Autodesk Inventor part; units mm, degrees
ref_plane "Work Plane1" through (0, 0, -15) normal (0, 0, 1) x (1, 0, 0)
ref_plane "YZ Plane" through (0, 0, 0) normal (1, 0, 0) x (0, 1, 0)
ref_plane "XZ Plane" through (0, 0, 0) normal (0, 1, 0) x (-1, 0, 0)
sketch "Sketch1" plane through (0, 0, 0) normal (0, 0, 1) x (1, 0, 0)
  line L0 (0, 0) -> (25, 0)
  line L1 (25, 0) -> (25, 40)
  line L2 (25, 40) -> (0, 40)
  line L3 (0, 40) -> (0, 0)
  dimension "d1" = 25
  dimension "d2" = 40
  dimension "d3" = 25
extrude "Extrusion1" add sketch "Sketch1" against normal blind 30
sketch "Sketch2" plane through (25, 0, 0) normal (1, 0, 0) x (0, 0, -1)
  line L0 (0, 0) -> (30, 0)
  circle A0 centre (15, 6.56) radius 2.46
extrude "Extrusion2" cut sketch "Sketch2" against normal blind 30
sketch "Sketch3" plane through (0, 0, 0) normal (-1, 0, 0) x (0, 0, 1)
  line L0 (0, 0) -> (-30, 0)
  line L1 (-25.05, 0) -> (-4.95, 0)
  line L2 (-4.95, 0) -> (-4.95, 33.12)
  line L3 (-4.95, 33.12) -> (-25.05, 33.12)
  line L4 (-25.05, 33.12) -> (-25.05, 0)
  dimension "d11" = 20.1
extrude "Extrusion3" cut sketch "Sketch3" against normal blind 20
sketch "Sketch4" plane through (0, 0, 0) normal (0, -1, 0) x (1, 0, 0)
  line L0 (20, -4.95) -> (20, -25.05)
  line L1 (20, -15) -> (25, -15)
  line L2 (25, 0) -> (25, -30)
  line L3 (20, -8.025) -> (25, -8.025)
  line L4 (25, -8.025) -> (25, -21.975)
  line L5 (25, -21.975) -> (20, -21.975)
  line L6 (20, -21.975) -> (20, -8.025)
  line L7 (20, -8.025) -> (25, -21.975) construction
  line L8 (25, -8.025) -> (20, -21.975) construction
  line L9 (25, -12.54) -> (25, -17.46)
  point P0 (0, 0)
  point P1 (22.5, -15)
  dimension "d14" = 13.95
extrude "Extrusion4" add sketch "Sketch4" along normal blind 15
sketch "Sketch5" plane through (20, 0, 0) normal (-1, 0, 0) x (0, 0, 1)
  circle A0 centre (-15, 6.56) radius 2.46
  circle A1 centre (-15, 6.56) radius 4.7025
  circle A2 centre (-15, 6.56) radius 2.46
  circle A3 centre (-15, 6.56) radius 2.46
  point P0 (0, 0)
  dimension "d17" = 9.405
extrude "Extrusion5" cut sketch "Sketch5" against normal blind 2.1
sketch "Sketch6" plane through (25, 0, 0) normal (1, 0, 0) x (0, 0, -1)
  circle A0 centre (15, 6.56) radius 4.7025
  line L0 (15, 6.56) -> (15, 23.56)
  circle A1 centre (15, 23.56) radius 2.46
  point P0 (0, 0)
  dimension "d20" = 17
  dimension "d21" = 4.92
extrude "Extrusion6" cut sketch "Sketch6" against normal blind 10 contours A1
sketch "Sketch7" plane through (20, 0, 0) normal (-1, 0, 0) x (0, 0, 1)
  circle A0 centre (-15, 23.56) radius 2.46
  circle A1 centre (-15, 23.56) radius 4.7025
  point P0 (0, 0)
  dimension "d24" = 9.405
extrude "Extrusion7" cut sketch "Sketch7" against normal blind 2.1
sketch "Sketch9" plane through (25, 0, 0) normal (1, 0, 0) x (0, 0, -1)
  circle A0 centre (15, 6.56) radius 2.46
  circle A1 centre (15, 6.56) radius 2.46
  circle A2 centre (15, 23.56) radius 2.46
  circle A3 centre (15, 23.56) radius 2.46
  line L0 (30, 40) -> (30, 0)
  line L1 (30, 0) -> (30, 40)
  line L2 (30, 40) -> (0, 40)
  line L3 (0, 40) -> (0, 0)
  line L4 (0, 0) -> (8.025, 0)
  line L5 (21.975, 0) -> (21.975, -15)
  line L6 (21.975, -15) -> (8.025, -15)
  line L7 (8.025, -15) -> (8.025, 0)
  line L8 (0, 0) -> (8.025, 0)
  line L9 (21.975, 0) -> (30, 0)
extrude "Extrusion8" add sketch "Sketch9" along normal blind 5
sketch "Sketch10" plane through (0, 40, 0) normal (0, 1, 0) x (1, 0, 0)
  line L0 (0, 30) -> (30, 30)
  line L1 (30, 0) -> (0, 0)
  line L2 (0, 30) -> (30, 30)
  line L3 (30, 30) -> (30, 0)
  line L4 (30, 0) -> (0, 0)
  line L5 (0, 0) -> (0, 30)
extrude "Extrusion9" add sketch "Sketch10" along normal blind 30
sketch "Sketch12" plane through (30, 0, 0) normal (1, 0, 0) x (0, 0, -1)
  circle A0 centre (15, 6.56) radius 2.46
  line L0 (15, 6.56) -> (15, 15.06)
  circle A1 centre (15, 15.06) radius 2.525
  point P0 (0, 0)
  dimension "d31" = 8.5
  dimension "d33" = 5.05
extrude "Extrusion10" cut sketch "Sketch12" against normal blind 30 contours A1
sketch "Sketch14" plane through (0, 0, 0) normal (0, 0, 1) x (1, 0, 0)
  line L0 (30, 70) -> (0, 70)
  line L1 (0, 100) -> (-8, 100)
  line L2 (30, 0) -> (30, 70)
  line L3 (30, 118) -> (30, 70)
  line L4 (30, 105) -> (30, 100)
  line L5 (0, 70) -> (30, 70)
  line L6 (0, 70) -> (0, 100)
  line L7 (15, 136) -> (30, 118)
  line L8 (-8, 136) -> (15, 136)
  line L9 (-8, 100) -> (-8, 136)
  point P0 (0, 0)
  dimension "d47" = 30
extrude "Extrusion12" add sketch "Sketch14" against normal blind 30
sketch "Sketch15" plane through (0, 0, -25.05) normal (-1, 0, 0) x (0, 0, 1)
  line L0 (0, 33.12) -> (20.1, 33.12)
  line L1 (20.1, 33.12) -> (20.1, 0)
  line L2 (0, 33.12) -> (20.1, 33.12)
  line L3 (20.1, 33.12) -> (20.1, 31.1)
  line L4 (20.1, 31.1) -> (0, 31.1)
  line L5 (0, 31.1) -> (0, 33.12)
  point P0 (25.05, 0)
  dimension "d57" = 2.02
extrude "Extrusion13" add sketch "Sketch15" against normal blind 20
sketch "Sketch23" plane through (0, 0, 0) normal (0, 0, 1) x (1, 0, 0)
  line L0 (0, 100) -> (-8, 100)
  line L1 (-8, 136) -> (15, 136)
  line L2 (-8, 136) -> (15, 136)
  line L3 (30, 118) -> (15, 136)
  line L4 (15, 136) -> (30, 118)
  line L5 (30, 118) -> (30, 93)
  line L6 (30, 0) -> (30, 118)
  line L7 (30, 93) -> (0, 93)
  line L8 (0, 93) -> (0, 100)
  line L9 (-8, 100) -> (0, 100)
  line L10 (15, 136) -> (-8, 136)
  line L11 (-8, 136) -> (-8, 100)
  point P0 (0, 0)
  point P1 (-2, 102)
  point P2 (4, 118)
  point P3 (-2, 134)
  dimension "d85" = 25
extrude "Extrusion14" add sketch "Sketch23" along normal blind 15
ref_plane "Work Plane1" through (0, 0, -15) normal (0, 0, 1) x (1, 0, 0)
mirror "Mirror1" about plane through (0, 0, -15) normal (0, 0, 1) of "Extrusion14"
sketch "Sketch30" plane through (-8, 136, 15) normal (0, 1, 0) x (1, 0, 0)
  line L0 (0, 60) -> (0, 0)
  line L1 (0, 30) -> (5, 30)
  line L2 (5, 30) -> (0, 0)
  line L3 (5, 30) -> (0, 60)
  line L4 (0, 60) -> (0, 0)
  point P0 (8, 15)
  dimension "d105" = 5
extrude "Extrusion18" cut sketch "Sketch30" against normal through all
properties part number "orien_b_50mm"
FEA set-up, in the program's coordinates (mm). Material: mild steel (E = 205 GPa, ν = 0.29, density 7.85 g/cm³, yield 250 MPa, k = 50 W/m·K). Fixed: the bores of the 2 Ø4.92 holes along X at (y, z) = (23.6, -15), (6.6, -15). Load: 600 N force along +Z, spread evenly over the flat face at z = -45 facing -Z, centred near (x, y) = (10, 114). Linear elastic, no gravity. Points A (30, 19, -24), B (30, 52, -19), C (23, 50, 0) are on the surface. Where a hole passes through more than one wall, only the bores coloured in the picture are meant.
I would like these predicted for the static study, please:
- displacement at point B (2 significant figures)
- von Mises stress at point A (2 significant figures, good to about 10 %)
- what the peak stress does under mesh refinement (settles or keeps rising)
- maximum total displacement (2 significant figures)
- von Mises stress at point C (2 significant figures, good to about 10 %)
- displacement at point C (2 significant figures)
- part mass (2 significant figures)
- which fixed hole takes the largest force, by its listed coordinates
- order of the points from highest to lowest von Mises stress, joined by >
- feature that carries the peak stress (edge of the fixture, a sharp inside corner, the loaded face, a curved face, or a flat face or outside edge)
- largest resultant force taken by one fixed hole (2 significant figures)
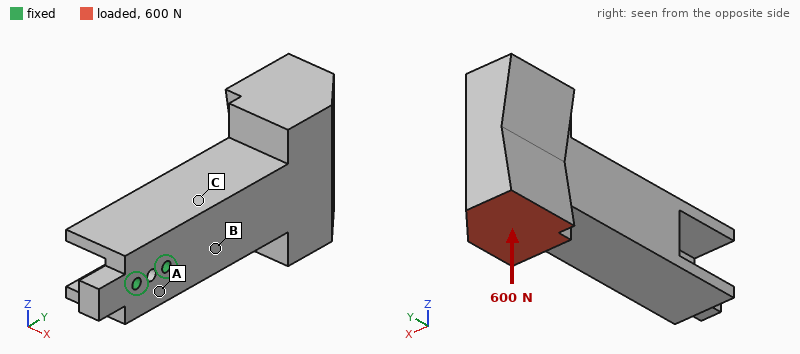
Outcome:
8.0 µm
18 MPa
keeps rising
46 µm
9.6 MPa
9.4 µm
1.2 kg
(23.6, -15)
A > C > B
edge of the fixture
2.9 kN
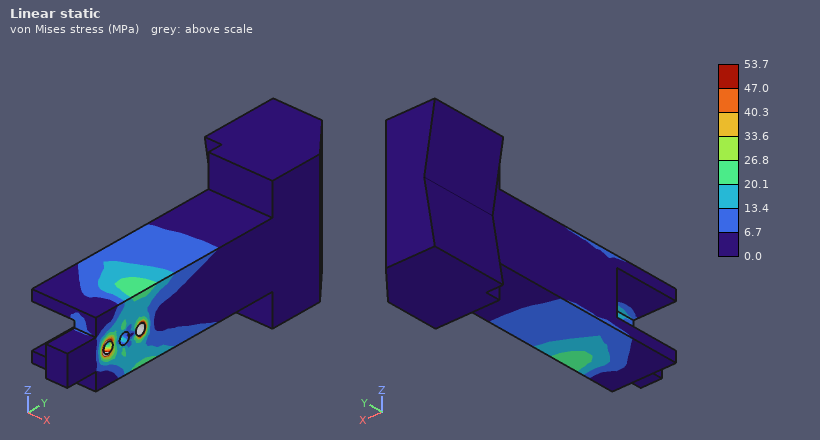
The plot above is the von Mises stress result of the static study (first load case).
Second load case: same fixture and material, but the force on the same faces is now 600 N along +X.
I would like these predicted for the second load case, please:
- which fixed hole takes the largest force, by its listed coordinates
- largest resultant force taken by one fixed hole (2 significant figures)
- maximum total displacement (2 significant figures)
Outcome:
(23.6, -15)
2.8 kN
73 µm
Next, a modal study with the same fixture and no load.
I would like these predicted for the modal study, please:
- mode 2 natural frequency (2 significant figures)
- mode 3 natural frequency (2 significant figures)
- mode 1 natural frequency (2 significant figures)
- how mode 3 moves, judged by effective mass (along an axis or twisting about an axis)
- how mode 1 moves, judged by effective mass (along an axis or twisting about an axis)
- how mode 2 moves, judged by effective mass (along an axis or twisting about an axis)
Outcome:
770 Hz
1900 Hz
660 Hz
twisting about Y
along X
along Z
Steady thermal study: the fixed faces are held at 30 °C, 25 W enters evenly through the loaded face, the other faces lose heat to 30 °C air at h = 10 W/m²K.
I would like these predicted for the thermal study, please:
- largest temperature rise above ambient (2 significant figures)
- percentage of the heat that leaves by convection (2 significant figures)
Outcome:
56 K
27 %
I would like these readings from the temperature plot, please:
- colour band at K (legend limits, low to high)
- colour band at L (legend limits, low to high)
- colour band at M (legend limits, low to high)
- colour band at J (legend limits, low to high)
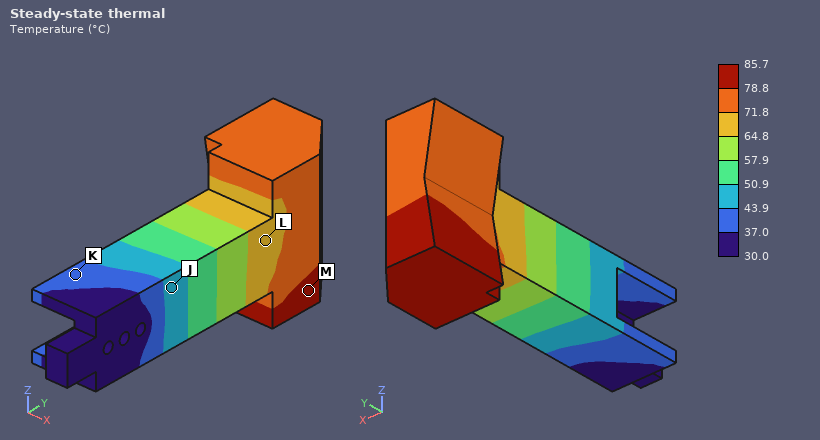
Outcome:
37.0 to 43.9 °C
64.8 to 71.8 °C
78.8 to 85.7 °C
43.9 to 50.9 °C
